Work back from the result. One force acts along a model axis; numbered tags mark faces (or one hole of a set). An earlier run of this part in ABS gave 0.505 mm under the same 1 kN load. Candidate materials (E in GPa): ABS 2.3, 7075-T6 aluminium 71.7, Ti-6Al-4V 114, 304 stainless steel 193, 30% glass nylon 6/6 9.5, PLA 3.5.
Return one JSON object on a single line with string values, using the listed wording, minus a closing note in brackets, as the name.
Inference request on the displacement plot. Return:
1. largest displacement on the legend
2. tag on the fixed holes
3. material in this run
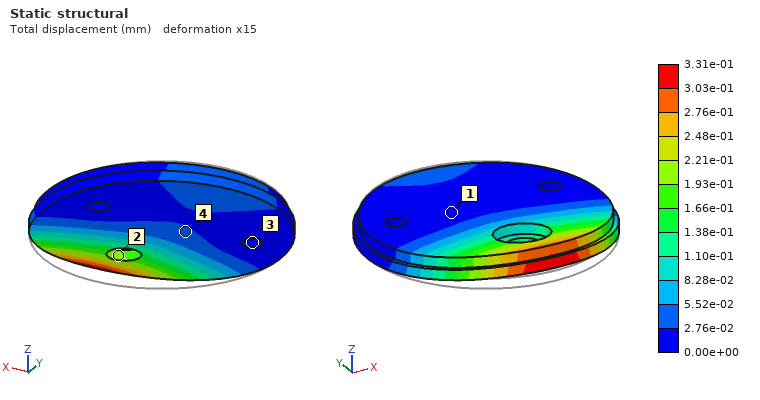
{"largest displacement on the legend": "3.31e-01 mm", "tag on the fixed holes": "3", "material in this run": "PLA"}
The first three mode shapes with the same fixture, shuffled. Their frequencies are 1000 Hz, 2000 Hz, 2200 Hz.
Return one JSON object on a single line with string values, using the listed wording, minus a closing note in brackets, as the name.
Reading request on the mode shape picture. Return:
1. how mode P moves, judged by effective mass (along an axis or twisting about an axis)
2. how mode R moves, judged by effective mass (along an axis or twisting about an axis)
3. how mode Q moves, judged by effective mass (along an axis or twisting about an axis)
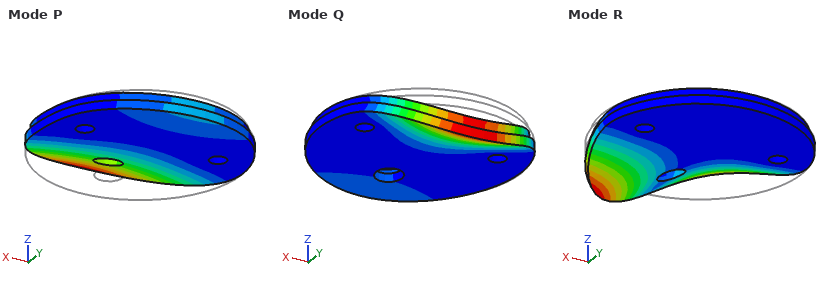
{"how mode P moves, judged by effective mass": "along Z", "how mode R moves, judged by effective mass": "twisting about Y", "how mode Q moves, judged by effective mass": "along Z"}
